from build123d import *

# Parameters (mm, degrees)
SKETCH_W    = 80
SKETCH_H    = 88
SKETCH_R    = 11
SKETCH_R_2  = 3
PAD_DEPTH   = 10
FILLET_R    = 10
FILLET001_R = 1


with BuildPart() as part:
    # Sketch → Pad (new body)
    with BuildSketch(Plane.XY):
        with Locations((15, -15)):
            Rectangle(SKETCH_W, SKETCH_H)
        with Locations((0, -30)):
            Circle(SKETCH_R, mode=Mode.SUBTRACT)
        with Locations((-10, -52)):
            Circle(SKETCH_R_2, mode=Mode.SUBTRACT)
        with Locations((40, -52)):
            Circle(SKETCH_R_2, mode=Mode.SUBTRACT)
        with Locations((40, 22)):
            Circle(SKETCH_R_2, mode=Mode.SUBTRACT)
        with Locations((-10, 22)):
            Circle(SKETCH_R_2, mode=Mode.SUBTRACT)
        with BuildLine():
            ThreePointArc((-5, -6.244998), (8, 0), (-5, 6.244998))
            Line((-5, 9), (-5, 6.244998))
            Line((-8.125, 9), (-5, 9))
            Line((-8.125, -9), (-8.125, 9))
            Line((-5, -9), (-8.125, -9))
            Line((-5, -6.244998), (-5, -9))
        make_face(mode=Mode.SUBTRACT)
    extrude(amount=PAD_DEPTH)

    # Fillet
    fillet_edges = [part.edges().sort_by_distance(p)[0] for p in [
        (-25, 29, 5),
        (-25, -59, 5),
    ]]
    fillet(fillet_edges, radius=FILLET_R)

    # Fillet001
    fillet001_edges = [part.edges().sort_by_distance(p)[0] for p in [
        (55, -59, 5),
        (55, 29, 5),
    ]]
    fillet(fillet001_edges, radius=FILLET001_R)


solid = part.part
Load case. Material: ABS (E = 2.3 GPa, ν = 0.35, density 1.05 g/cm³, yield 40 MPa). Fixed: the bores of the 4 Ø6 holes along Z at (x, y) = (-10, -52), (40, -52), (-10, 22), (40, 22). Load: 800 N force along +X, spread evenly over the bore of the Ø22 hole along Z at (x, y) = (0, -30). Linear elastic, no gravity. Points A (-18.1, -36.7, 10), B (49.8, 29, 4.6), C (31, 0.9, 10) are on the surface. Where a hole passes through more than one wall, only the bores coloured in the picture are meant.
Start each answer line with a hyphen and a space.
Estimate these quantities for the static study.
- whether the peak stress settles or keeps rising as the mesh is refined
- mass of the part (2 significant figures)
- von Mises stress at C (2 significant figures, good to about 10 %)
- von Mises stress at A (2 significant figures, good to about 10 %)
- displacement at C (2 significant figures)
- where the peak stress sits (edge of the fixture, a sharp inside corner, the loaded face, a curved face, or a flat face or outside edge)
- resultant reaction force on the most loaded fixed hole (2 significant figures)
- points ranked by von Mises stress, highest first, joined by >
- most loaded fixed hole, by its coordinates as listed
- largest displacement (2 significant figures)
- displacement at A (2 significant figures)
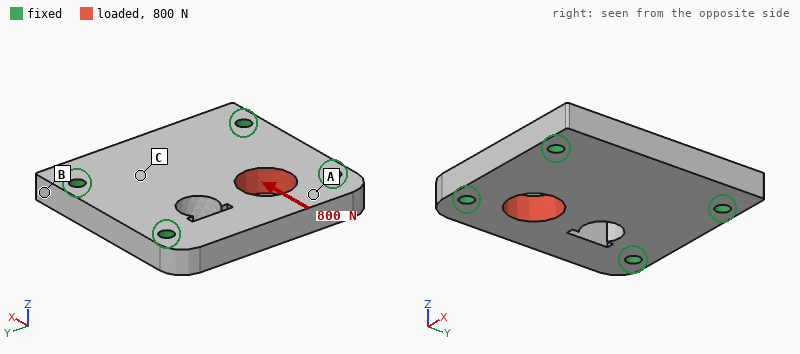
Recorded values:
- keeps rising
- 66 g
- 0.88 MPa
- 1.6 MPa
- 13 µm
- edge of the fixture
- 330 N
- A > C > B
- (-10, -52)
- 43 µm
- 29 µm
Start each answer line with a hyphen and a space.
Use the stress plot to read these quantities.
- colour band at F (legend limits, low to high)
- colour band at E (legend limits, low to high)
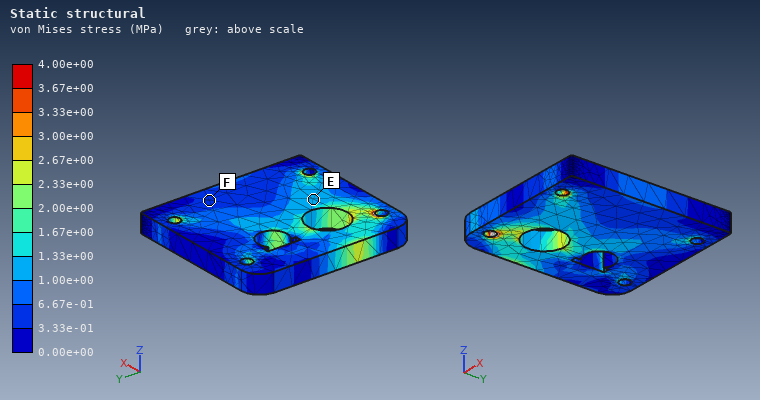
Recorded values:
- 3.33e-01 to 6.67e-01 MPa
- 1.00e+00 to 1.33e+00 MPa
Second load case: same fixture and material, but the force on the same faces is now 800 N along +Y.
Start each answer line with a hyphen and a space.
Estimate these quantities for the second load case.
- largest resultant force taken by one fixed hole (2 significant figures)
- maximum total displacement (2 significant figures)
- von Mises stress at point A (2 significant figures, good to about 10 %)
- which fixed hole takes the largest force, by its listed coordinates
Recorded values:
- 370 N
- 28 µm
- 0.87 MPa
- (-10, -52)
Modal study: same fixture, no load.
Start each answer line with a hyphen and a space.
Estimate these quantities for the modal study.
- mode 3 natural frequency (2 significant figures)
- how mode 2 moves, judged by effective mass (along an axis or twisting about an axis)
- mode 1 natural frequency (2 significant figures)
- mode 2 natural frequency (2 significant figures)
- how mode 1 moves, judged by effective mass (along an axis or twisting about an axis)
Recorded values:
- 3400 Hz
- twisting about Y
- 2100 Hz
- 2600 Hz
- along Z
